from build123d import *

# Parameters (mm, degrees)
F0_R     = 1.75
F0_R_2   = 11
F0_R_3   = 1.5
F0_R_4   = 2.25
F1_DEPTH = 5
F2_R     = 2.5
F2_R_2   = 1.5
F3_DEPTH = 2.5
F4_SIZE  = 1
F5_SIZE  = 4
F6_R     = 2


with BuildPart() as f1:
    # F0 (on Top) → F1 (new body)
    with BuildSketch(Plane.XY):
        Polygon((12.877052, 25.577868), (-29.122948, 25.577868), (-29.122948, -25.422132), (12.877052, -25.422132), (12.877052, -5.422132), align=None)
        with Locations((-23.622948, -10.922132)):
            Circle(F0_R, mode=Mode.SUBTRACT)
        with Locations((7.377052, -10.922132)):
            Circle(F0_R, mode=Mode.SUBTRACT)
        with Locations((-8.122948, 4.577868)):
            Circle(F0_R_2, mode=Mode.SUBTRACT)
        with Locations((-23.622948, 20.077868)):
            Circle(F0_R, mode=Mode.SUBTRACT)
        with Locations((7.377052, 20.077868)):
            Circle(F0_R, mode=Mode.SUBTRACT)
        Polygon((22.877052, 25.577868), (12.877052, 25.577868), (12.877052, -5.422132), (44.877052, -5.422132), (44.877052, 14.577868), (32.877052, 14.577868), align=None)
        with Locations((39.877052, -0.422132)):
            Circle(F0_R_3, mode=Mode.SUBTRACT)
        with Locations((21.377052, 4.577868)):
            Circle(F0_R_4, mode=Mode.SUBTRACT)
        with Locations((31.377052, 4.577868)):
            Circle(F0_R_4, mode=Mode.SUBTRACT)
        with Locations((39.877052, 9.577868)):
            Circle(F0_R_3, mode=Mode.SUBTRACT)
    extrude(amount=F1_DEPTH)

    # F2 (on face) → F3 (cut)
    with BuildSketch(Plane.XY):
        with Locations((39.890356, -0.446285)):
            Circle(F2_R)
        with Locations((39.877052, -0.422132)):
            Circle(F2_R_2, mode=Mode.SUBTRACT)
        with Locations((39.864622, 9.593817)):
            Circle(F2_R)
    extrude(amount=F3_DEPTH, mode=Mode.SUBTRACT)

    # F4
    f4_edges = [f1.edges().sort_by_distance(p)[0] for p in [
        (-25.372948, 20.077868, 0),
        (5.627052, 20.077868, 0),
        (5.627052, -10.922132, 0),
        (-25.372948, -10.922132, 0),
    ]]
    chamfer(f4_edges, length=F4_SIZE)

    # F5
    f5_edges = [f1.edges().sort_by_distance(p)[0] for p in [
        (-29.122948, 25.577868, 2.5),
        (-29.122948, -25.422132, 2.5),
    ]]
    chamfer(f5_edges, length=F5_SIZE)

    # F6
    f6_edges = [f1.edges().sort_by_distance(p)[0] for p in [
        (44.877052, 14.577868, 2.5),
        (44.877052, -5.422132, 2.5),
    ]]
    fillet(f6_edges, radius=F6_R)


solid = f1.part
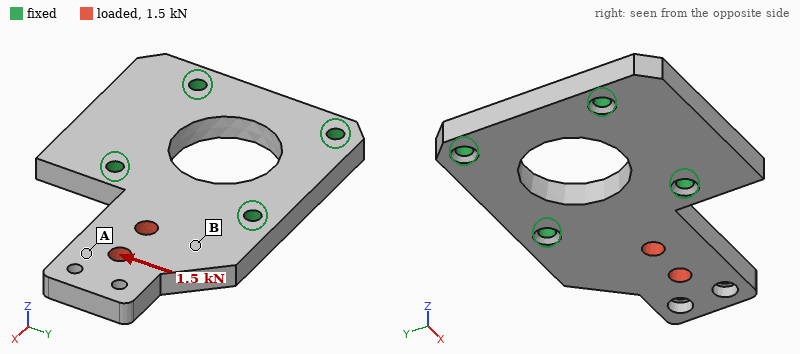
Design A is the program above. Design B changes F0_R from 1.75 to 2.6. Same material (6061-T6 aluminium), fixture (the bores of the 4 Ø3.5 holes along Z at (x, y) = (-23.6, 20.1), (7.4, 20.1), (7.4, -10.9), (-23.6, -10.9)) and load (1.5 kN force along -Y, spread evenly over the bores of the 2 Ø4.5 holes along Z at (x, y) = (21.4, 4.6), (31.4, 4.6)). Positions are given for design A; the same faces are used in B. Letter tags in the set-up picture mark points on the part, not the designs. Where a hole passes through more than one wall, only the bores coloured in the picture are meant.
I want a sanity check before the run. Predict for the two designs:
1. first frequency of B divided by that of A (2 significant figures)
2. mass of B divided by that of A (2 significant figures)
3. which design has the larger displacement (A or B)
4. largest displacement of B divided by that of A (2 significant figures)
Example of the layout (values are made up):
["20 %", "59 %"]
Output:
["1.1", "0.98", "A", "0.90"]
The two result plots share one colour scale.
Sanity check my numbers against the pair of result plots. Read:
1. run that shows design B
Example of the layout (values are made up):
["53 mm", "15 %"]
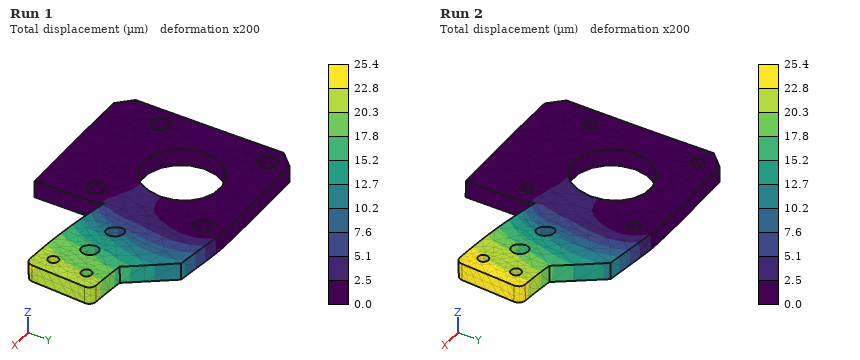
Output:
["Run 1"]
